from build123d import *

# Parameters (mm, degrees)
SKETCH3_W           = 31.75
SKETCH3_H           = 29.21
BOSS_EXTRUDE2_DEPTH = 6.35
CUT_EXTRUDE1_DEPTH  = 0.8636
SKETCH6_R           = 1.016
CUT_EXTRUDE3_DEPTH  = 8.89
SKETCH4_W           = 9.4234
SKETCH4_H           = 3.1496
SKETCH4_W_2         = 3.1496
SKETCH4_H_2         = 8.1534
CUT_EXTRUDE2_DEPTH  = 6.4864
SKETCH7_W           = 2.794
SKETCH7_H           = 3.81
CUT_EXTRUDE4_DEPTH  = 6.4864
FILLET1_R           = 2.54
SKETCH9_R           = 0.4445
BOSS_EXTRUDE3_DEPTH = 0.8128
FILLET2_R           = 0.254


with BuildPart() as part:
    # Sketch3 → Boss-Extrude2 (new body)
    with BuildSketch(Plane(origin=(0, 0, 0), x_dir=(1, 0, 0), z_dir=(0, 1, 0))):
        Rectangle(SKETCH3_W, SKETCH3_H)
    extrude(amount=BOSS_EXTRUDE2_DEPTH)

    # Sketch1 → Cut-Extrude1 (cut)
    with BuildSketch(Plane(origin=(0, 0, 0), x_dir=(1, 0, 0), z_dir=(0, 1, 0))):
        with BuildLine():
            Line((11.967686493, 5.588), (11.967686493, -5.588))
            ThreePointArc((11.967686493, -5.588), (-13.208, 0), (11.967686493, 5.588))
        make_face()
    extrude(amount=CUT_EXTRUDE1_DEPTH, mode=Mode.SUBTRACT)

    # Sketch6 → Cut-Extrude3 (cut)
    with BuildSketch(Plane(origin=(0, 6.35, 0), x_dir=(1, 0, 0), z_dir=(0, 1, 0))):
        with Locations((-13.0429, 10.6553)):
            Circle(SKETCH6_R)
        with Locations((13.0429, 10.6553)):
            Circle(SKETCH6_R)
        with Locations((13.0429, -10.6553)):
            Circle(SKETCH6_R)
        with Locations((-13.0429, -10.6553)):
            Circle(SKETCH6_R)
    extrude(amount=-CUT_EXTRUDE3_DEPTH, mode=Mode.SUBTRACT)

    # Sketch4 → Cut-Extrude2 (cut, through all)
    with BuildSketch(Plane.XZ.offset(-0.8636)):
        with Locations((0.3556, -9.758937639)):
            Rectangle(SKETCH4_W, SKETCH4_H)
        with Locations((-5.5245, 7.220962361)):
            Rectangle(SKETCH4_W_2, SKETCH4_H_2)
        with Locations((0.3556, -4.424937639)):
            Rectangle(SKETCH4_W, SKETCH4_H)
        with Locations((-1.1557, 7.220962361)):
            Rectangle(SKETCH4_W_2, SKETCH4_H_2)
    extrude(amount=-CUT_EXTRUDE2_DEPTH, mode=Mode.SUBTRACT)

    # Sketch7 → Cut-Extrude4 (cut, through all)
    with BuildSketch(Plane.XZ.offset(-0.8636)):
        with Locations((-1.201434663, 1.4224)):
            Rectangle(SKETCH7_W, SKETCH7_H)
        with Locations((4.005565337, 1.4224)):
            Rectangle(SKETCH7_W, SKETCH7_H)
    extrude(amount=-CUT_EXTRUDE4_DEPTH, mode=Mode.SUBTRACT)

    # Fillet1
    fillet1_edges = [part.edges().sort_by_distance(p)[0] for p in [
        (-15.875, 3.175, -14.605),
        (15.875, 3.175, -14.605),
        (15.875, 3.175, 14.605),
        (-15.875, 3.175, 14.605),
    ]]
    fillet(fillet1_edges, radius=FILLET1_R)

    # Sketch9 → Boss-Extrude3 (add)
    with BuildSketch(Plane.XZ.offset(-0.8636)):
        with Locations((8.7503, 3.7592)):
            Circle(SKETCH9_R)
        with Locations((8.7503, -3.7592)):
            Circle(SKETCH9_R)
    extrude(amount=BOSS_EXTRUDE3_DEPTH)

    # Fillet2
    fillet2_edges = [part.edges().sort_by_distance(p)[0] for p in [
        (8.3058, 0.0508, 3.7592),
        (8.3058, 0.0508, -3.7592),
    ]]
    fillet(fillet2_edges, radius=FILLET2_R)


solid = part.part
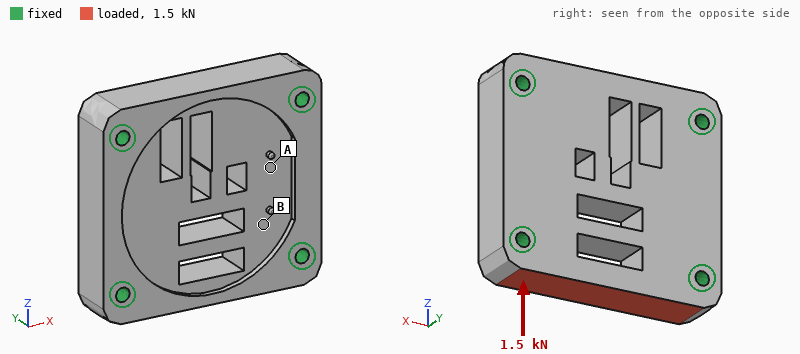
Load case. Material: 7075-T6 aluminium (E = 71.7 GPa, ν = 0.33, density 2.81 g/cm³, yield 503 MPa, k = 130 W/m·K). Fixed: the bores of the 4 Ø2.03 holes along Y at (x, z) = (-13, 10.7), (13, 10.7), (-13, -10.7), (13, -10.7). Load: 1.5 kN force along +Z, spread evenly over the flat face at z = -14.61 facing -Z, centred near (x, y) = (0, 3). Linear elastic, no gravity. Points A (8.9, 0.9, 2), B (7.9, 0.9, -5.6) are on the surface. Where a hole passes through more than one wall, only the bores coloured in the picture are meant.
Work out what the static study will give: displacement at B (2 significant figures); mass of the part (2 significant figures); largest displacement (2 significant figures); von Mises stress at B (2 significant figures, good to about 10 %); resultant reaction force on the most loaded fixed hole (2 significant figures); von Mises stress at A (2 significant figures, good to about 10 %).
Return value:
1.6 µm
13 g
10 µm
14 MPa
530 N
6.7 MPa
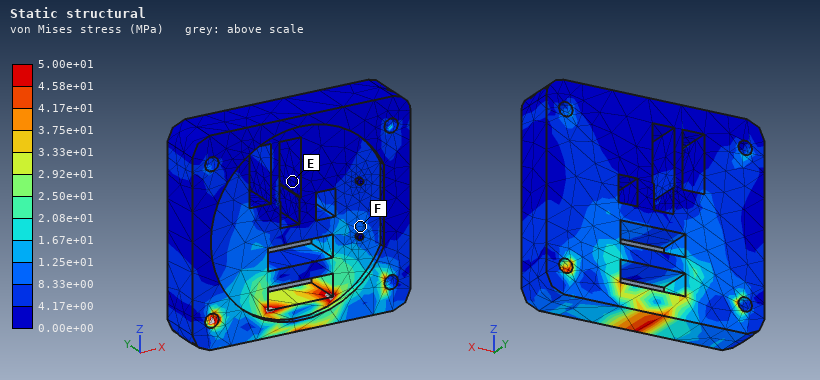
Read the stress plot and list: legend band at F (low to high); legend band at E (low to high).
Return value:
8.33e+00 to 1.25e+01 MPa
0.00e+00 to 4.17e+00 MPa
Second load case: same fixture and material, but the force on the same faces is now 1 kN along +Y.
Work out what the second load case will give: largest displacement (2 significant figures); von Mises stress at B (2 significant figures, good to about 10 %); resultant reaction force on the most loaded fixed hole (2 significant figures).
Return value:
16 µm
14 MPa
530 N
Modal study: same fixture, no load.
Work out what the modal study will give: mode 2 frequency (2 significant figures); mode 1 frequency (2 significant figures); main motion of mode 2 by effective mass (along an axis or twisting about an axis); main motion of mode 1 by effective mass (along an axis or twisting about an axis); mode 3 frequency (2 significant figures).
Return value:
39 kHz
28 kHz
twisting about X
along Y
43 kHz
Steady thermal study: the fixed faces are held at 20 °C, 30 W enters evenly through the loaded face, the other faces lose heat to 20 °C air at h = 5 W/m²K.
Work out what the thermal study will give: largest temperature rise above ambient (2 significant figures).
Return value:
23 K
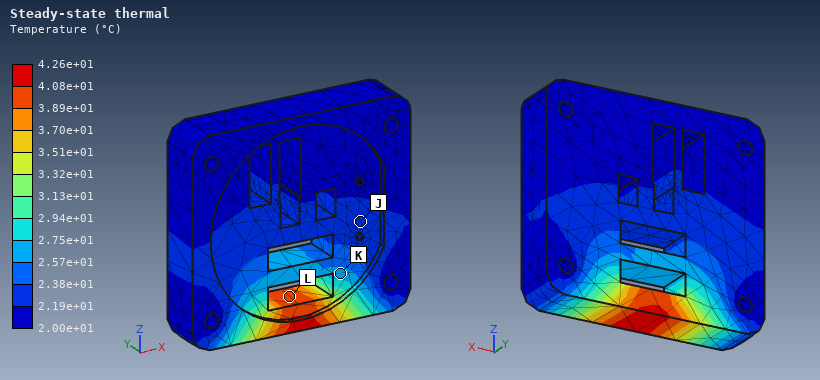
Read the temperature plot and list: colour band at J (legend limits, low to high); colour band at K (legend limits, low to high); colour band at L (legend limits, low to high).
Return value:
2.19e+01 to 2.38e+01 °C
2.57e+01 to 2.75e+01 °C
3.89e+01 to 4.08e+01 °C
